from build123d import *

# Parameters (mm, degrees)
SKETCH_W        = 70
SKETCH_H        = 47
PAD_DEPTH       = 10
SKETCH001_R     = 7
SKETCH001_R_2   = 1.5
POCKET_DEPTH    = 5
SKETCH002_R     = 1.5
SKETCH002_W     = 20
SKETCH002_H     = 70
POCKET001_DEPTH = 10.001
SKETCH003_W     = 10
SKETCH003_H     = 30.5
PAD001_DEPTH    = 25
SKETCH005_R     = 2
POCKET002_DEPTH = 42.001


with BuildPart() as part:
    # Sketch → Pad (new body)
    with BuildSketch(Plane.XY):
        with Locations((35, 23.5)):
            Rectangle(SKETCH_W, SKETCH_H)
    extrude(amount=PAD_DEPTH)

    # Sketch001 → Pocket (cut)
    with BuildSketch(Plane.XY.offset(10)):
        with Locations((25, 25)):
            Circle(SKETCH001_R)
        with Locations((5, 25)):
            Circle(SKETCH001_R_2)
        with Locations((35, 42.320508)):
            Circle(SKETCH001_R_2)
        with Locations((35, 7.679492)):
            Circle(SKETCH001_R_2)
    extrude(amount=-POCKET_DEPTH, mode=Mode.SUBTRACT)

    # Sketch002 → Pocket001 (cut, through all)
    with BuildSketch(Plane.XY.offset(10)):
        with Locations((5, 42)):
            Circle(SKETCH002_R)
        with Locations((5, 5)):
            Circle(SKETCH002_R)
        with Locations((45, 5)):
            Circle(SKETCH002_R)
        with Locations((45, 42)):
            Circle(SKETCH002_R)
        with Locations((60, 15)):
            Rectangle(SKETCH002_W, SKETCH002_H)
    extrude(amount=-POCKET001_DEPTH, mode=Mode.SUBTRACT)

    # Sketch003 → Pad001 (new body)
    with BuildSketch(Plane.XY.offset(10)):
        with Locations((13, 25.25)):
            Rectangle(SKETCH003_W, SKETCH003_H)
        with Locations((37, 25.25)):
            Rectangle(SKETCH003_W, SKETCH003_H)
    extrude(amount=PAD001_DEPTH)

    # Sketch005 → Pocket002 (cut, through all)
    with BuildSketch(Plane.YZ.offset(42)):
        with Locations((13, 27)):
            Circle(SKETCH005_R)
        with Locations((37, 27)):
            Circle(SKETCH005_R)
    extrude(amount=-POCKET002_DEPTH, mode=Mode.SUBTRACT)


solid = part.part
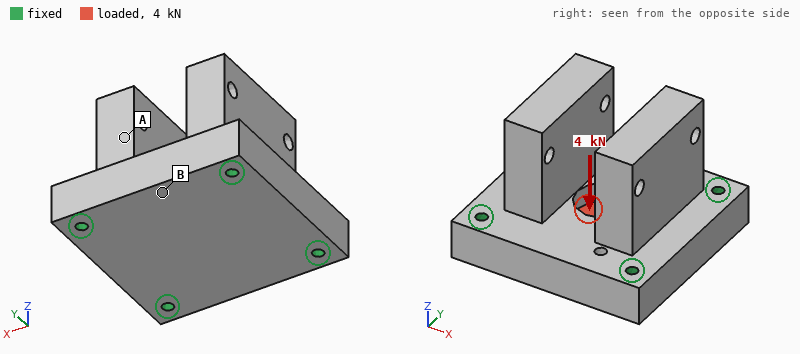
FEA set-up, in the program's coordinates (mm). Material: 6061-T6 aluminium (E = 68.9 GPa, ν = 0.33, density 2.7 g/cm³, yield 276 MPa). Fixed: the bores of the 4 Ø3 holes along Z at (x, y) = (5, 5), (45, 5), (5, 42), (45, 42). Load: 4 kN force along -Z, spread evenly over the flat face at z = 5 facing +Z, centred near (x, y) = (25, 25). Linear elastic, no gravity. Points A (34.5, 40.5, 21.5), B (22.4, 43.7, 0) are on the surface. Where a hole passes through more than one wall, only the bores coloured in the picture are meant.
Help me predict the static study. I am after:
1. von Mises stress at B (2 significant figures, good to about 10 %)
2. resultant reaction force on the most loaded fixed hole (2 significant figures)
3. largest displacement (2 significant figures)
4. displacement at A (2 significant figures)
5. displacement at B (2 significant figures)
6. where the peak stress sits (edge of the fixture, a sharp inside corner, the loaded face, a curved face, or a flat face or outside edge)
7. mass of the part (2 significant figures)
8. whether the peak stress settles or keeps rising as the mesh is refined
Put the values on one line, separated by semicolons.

20 MPa; 1.1 kN; 26 µm; 16 µm; 9.7 µm; edge of the fixture; 100 g; keeps rising
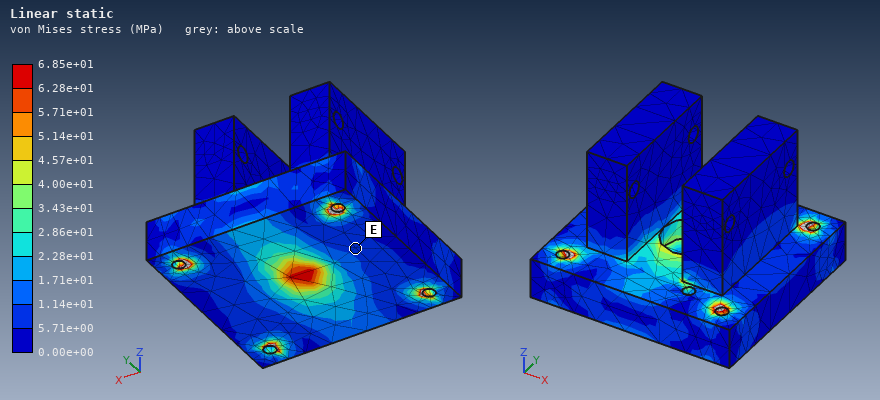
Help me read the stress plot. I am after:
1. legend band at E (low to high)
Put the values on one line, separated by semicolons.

5.71e+00 to 1.14e+01 MPa
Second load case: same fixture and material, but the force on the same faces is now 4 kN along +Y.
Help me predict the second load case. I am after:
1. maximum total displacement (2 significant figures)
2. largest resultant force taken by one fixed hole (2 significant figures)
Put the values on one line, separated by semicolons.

8.2 µm; 1.1 kN
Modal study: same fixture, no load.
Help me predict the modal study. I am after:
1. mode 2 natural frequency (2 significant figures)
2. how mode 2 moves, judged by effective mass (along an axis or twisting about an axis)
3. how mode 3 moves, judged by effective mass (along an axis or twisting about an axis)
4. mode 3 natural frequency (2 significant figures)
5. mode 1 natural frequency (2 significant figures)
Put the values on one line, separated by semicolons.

8900 Hz; along X; along Y; 13 kHz; 7400 Hz
